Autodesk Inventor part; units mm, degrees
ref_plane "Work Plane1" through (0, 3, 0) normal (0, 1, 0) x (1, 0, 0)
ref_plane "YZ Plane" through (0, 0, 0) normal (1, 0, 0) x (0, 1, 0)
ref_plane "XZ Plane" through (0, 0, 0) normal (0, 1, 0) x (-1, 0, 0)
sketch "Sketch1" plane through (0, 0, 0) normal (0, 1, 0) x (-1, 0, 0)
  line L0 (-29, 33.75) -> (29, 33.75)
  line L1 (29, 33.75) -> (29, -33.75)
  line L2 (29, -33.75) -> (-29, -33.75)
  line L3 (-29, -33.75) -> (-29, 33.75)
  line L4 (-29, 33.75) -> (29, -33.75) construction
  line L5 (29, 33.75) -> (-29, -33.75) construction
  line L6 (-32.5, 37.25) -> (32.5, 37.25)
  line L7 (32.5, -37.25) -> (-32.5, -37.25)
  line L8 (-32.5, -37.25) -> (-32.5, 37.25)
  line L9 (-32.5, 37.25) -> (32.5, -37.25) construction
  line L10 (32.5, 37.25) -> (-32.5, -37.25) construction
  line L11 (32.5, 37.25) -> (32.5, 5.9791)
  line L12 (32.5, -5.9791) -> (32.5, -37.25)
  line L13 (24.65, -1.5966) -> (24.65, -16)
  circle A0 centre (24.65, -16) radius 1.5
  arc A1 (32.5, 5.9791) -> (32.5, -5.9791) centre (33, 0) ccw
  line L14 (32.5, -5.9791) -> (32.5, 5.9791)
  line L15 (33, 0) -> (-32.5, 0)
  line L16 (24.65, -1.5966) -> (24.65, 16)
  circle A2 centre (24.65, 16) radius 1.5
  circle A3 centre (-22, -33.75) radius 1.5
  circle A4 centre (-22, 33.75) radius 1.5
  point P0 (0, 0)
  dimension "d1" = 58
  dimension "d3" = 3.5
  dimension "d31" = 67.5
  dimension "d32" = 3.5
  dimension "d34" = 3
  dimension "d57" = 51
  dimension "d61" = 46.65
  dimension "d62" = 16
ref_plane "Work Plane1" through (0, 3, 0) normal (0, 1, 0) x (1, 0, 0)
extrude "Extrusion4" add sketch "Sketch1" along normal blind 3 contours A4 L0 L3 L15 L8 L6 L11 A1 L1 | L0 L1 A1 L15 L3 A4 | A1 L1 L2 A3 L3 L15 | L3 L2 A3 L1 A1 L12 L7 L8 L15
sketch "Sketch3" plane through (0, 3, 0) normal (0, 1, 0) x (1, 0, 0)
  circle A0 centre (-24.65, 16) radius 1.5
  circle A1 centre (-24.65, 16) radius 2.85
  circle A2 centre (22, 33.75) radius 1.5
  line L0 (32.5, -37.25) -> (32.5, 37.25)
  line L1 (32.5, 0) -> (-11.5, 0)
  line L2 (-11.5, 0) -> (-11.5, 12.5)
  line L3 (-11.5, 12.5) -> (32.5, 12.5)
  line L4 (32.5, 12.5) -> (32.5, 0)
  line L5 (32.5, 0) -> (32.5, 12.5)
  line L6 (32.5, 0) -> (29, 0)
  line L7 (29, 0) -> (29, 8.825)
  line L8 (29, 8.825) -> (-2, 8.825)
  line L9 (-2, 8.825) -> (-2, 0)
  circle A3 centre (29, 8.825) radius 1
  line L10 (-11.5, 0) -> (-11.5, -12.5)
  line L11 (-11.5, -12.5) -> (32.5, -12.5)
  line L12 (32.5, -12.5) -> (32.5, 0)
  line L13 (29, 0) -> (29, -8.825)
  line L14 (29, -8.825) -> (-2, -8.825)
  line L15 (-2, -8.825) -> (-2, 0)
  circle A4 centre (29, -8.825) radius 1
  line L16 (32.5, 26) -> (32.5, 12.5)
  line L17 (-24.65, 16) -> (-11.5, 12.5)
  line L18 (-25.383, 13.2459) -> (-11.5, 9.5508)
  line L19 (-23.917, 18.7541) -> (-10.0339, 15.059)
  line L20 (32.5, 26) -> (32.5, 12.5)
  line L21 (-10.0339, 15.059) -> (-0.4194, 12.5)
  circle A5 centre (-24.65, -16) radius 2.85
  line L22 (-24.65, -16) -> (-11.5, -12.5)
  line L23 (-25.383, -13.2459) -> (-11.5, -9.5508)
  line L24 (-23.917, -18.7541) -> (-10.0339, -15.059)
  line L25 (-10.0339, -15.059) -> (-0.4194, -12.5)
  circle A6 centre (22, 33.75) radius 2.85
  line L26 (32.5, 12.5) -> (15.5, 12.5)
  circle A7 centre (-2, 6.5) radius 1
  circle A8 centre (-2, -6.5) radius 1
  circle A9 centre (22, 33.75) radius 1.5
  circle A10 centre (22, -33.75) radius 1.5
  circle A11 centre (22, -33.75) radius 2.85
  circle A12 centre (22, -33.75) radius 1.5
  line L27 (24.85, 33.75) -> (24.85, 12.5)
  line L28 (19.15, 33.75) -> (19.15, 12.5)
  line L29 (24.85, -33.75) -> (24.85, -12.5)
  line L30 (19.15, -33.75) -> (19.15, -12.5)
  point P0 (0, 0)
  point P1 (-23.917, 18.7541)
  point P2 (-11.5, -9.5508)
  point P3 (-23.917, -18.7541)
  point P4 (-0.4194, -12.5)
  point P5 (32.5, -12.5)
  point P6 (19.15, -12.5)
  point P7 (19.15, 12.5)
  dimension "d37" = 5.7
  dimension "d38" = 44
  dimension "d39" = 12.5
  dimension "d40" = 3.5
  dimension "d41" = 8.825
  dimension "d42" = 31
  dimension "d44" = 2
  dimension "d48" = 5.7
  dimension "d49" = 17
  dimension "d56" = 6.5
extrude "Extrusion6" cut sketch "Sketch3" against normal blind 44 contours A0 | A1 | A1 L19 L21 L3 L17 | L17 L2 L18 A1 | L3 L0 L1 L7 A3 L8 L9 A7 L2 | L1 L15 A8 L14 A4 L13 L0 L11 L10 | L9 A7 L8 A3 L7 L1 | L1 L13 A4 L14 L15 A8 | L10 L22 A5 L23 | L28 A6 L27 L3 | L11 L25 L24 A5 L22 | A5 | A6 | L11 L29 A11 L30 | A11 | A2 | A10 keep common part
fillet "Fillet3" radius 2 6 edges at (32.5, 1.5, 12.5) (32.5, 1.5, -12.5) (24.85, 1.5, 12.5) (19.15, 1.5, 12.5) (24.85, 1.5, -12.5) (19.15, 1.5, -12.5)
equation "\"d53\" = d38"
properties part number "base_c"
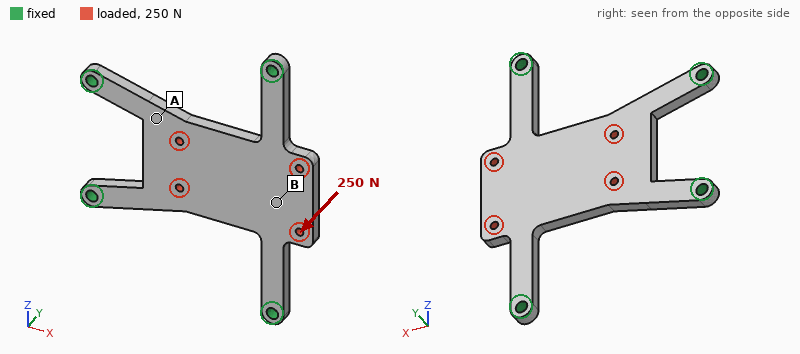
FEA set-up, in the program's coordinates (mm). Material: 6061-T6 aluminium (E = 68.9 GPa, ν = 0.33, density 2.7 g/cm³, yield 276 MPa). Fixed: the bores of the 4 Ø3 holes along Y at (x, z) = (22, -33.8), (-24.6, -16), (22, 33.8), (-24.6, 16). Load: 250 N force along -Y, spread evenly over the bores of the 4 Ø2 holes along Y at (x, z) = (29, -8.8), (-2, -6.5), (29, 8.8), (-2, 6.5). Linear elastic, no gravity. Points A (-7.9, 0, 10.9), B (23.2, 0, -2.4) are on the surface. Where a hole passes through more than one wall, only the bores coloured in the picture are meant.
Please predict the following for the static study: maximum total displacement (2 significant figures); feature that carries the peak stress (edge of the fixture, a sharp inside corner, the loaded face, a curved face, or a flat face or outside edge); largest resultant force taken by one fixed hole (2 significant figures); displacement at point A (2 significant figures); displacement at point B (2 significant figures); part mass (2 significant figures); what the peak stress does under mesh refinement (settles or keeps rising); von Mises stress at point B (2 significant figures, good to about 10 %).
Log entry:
0.20 mm
edge of the fixture
87 N
0.050 mm
0.15 mm
12 g
keeps rising
33 MPa
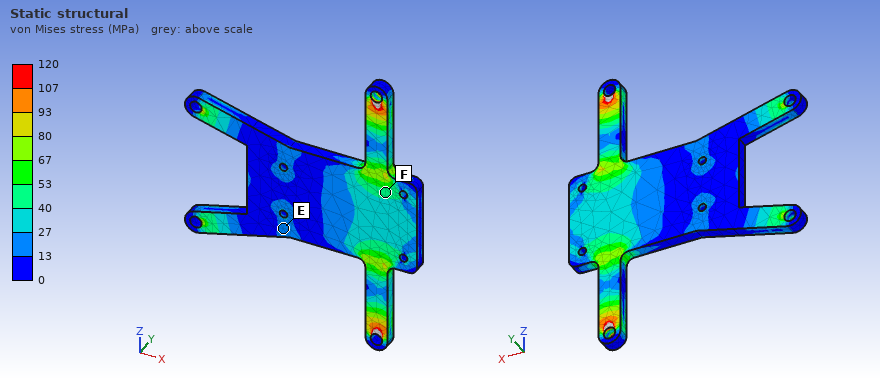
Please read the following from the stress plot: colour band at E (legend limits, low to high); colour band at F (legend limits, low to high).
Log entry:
13 to 27 MPa
40 to 53 MPa
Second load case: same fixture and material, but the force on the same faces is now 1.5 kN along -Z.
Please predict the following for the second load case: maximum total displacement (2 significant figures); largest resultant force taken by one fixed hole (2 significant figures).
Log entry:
27 µm
550 N
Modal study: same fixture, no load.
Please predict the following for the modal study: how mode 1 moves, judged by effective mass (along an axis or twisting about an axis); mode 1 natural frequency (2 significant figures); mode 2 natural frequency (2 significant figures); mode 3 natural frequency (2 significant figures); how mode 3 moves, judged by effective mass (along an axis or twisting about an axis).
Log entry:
along Y
2400 Hz
4600 Hz
7000 Hz
twisting about X
